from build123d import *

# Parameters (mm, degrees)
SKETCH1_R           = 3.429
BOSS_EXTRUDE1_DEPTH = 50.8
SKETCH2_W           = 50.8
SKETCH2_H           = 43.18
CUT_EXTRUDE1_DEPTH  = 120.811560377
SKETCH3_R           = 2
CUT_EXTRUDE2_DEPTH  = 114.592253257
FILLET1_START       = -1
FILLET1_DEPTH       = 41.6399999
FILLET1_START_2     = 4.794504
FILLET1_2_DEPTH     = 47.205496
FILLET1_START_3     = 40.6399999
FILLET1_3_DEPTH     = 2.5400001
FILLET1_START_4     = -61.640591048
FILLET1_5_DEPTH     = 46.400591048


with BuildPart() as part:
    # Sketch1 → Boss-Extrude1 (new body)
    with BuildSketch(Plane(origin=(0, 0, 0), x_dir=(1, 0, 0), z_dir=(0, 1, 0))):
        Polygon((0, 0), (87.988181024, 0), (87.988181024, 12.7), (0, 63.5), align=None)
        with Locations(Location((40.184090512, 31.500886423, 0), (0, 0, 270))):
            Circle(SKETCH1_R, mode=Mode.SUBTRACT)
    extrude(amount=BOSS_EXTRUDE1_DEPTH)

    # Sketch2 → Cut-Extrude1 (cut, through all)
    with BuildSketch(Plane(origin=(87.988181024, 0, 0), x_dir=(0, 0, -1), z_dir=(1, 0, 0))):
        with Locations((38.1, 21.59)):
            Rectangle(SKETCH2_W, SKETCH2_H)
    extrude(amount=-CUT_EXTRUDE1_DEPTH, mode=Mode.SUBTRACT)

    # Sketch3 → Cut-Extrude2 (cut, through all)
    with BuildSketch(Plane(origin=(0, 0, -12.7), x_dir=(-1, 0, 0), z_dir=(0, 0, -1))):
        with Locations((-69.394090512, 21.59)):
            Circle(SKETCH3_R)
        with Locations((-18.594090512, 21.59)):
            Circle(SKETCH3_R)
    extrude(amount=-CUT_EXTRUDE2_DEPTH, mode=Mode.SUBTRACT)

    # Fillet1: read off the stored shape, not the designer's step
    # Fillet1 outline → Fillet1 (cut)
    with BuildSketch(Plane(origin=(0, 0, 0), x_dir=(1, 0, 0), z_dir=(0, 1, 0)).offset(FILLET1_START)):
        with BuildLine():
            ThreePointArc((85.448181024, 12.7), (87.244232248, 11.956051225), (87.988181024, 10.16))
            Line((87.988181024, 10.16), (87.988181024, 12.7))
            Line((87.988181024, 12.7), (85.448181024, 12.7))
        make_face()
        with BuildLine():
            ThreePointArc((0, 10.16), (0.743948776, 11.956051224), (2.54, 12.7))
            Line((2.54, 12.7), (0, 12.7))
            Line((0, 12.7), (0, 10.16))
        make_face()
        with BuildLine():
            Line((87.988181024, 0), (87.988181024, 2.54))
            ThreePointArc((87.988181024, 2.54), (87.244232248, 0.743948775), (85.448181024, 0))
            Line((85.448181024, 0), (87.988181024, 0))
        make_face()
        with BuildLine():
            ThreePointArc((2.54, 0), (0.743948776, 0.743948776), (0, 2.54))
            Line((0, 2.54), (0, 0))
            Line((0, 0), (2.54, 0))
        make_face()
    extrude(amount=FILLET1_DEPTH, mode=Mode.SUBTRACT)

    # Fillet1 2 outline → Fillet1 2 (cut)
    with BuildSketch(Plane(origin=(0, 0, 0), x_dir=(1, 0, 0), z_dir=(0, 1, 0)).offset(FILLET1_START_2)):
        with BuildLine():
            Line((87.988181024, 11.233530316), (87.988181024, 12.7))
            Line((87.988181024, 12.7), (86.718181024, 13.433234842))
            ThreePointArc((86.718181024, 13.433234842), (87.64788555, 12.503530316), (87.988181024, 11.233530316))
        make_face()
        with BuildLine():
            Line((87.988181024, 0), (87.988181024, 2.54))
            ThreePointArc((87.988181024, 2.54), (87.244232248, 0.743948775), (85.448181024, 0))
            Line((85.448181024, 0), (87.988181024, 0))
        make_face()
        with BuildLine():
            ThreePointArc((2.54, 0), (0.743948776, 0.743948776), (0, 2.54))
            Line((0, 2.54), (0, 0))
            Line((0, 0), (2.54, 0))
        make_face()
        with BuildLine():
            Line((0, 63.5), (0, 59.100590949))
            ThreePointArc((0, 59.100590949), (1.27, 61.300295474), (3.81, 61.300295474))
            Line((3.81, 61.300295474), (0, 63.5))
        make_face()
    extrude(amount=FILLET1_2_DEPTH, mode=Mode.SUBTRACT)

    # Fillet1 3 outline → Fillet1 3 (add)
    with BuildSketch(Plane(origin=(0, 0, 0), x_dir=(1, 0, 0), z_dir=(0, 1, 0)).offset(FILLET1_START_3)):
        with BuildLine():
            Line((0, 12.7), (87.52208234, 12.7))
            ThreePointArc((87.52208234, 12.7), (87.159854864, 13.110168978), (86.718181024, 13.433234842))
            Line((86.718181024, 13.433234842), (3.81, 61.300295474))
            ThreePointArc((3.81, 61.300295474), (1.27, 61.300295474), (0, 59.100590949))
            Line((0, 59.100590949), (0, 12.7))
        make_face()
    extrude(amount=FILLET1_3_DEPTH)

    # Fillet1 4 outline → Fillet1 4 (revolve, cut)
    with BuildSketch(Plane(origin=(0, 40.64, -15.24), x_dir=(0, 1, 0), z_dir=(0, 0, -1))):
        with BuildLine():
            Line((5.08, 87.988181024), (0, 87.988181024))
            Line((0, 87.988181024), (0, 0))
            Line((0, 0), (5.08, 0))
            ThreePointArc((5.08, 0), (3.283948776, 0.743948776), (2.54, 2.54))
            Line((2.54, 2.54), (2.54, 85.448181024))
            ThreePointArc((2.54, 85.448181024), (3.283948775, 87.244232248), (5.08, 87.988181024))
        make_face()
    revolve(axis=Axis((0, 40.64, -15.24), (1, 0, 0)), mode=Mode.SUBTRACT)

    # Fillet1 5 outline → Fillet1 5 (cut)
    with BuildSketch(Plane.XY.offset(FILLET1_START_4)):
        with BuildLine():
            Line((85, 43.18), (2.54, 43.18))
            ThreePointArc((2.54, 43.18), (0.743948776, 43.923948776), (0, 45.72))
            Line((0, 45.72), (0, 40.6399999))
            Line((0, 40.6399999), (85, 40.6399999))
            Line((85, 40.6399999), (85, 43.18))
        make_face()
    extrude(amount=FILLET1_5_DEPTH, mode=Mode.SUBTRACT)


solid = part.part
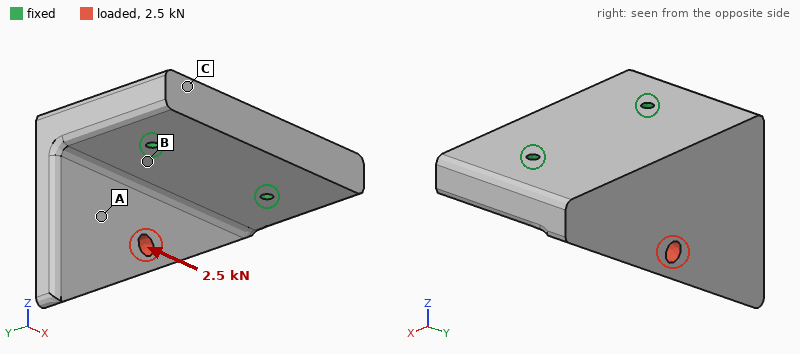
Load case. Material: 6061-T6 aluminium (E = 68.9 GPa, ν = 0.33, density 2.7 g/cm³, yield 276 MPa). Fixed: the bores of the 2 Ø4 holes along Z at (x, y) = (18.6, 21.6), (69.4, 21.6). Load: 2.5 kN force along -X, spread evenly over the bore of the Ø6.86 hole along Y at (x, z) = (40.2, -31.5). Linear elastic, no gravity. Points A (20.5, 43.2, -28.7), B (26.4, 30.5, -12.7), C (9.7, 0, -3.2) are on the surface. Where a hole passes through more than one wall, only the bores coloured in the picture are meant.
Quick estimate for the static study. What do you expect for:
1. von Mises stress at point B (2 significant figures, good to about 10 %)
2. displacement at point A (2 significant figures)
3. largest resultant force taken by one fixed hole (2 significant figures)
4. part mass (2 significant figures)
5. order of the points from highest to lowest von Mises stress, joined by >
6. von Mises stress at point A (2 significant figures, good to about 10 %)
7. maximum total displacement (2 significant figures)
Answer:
17 MPa
24 µm
2.0 kN
200 g
B > A > C
9.5 MPa
52 µm
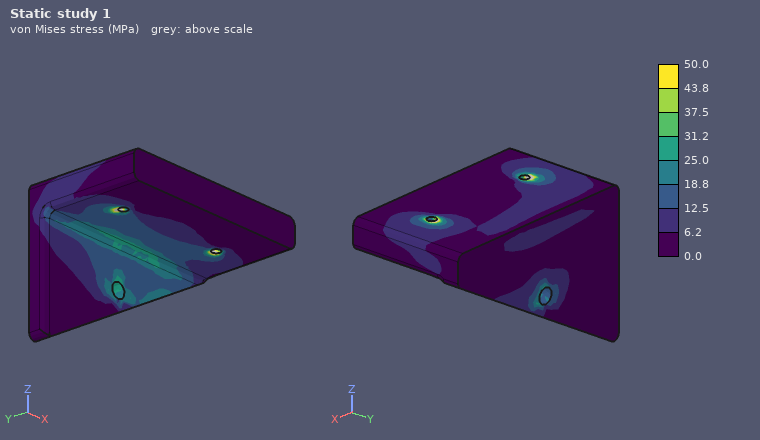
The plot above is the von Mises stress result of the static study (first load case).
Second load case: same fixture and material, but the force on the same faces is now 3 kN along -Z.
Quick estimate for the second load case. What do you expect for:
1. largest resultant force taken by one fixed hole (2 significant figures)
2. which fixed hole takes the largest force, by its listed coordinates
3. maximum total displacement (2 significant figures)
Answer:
1.7 kN
(18.6, 21.6)
0.10 mm
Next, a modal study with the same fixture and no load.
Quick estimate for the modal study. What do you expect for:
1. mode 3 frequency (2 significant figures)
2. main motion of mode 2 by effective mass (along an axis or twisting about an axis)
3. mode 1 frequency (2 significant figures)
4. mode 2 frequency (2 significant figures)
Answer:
5800 Hz
along Z
2700 Hz
5500 Hz
